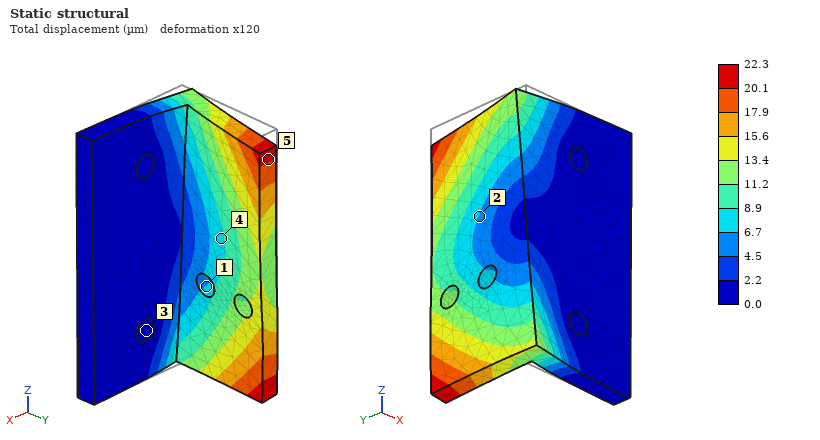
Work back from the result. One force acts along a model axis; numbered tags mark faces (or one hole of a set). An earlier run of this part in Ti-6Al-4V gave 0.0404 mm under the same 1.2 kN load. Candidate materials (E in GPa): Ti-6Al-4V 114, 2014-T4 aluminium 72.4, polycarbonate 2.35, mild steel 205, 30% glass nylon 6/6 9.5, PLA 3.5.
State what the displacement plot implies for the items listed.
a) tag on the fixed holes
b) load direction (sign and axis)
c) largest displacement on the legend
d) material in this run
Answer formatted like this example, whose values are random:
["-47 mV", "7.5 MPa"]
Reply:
["3", "-Z", "22.3 µm", "mild steel"]
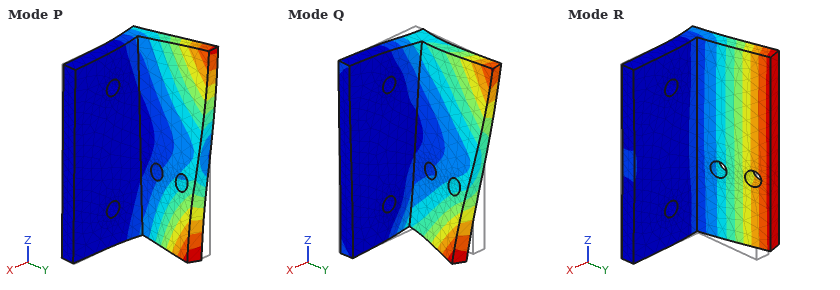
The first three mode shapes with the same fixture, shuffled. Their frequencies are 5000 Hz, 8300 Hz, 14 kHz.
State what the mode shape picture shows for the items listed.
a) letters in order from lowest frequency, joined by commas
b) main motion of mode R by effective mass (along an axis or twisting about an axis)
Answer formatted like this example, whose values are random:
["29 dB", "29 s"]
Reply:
["R, P, Q", "along X"]
